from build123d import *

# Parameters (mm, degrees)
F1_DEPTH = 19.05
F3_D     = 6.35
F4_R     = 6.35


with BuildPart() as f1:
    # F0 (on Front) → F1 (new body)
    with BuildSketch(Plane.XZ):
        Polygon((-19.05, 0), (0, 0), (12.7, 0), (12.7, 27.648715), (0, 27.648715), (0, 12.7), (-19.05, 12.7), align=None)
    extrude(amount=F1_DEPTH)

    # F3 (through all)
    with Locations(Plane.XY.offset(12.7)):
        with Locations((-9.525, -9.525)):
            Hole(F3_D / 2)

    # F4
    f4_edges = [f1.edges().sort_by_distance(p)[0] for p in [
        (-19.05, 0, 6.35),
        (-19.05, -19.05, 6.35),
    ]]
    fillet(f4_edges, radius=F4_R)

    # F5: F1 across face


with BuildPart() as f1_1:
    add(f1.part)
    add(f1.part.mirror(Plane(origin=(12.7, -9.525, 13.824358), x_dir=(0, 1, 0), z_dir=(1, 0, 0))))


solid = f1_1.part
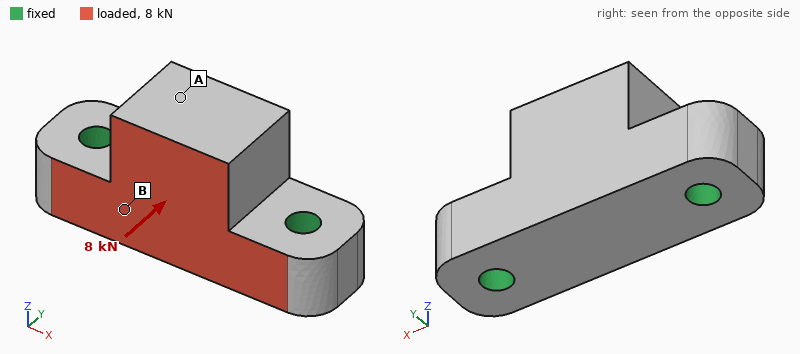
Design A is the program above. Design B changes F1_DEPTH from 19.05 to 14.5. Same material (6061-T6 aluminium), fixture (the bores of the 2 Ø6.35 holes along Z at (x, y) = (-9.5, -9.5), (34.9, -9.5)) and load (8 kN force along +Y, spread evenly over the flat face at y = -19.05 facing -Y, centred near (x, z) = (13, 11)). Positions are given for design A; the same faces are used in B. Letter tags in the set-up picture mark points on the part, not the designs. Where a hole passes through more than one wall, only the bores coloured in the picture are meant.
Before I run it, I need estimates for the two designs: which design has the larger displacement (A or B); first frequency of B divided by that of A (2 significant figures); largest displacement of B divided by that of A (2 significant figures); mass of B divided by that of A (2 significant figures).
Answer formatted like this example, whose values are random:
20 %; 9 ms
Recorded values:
B; 0.94; 1.5; 0.75
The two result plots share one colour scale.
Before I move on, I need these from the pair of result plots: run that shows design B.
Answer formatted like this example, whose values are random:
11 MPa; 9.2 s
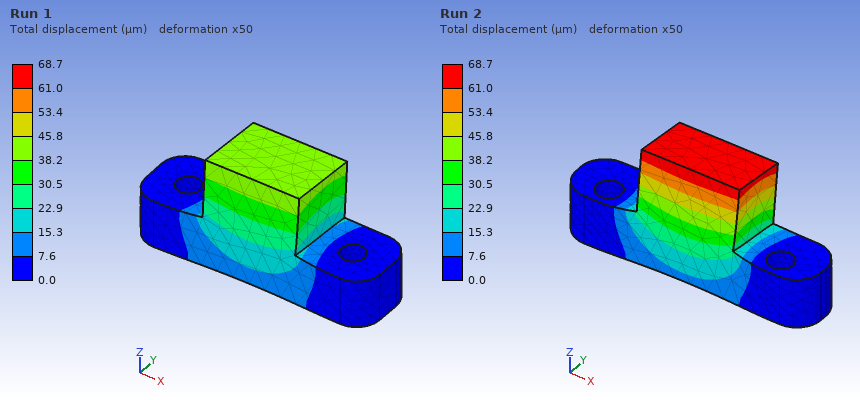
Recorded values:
Run 2
